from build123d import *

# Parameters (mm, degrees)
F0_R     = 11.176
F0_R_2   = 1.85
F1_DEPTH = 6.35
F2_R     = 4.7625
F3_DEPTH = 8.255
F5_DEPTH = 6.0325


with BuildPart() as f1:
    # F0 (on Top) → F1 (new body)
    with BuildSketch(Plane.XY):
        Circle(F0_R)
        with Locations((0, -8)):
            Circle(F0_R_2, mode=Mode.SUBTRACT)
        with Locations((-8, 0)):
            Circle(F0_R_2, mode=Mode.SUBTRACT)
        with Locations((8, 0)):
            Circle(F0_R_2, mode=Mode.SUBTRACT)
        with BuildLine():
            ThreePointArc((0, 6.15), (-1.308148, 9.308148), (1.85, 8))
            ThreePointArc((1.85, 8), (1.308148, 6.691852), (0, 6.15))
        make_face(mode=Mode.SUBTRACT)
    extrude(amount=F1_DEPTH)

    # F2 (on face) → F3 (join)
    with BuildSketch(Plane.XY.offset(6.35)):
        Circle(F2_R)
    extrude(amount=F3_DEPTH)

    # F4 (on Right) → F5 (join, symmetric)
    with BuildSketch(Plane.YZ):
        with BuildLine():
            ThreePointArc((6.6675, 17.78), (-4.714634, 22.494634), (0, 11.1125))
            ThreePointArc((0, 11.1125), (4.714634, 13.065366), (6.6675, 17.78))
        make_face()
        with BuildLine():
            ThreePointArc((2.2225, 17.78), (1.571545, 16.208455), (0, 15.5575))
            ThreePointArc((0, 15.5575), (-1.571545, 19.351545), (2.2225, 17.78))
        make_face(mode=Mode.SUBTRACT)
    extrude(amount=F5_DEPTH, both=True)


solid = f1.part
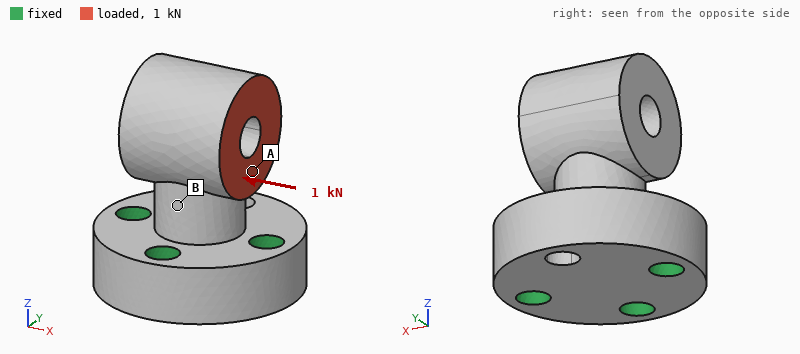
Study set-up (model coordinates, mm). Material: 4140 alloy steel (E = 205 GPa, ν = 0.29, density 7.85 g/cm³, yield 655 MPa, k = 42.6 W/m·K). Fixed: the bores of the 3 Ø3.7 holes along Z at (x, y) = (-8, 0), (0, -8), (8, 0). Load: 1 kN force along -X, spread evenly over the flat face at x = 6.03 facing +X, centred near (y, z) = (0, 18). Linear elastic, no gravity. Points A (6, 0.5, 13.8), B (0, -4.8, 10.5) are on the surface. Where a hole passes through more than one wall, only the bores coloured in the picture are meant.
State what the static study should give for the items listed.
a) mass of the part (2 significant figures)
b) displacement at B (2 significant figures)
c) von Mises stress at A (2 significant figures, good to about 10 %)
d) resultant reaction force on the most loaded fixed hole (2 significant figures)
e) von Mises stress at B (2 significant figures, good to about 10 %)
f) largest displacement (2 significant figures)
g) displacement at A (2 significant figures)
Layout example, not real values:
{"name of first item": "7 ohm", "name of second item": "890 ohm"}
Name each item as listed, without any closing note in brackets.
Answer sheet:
{"mass of the part": "32 g", "displacement at B": "3.5 µm", "von Mises stress at A": "15 MPa", "resultant reaction force on the most loaded fixed hole": "1.1 kN", "von Mises stress at B": "33 MPa", "largest displacement": "21 µm", "displacement at A": "9.6 µm"}
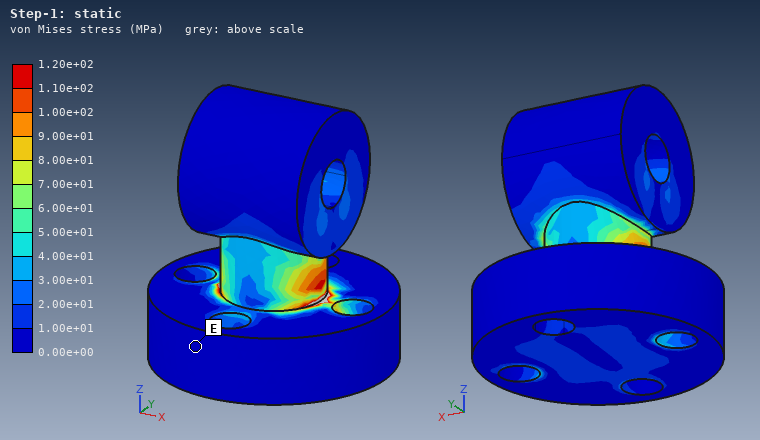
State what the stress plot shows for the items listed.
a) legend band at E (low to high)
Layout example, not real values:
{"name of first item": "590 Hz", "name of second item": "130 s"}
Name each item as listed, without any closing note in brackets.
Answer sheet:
{"legend band at E": "0.00e+00 to 1.00e+01 MPa"}
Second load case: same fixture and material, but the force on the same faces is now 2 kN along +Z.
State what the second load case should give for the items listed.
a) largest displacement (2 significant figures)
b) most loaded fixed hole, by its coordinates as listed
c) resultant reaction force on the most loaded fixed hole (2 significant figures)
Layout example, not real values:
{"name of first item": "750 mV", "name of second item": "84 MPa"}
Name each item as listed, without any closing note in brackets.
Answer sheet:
{"largest displacement": "28 µm", "most loaded fixed hole, by its coordinates as listed": "(8, 0)", "resultant reaction force on the most loaded fixed hole": "1.6 kN"}
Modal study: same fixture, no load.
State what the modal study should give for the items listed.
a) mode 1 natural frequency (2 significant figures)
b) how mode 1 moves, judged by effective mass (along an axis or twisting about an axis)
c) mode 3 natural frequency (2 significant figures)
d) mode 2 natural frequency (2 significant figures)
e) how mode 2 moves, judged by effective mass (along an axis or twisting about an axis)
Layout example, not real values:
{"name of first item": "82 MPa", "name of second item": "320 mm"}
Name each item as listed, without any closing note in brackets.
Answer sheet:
{"mode 1 natural frequency": "11 kHz", "how mode 1 moves, judged by effective mass": "along Y", "mode 3 natural frequency": "25 kHz", "mode 2 natural frequency": "12 kHz", "how mode 2 moves, judged by effective mass": "along X"}
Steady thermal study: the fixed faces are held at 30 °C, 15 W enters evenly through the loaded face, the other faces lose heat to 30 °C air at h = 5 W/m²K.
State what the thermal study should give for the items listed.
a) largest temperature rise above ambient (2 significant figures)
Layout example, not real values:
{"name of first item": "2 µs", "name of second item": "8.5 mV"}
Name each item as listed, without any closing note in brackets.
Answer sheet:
{"largest temperature rise above ambient": "75 K"}
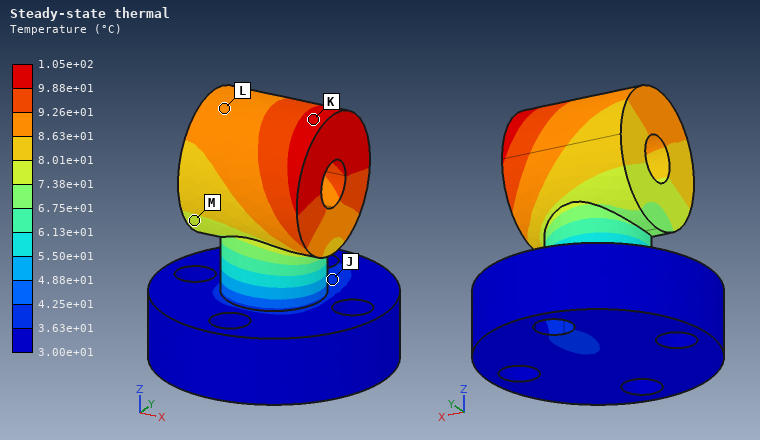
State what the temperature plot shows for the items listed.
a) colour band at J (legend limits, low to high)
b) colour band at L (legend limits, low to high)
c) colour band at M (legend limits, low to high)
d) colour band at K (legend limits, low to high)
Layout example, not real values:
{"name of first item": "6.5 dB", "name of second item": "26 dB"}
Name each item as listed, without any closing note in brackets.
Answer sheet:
{"colour band at J": "3.63e+01 to 4.25e+01 °C", "colour band at L": "8.63e+01 to 9.26e+01 °C", "colour band at M": "7.38e+01 to 8.01e+01 °C", "colour band at K": "9.88e+01 to 1.05e+02 °C"}
